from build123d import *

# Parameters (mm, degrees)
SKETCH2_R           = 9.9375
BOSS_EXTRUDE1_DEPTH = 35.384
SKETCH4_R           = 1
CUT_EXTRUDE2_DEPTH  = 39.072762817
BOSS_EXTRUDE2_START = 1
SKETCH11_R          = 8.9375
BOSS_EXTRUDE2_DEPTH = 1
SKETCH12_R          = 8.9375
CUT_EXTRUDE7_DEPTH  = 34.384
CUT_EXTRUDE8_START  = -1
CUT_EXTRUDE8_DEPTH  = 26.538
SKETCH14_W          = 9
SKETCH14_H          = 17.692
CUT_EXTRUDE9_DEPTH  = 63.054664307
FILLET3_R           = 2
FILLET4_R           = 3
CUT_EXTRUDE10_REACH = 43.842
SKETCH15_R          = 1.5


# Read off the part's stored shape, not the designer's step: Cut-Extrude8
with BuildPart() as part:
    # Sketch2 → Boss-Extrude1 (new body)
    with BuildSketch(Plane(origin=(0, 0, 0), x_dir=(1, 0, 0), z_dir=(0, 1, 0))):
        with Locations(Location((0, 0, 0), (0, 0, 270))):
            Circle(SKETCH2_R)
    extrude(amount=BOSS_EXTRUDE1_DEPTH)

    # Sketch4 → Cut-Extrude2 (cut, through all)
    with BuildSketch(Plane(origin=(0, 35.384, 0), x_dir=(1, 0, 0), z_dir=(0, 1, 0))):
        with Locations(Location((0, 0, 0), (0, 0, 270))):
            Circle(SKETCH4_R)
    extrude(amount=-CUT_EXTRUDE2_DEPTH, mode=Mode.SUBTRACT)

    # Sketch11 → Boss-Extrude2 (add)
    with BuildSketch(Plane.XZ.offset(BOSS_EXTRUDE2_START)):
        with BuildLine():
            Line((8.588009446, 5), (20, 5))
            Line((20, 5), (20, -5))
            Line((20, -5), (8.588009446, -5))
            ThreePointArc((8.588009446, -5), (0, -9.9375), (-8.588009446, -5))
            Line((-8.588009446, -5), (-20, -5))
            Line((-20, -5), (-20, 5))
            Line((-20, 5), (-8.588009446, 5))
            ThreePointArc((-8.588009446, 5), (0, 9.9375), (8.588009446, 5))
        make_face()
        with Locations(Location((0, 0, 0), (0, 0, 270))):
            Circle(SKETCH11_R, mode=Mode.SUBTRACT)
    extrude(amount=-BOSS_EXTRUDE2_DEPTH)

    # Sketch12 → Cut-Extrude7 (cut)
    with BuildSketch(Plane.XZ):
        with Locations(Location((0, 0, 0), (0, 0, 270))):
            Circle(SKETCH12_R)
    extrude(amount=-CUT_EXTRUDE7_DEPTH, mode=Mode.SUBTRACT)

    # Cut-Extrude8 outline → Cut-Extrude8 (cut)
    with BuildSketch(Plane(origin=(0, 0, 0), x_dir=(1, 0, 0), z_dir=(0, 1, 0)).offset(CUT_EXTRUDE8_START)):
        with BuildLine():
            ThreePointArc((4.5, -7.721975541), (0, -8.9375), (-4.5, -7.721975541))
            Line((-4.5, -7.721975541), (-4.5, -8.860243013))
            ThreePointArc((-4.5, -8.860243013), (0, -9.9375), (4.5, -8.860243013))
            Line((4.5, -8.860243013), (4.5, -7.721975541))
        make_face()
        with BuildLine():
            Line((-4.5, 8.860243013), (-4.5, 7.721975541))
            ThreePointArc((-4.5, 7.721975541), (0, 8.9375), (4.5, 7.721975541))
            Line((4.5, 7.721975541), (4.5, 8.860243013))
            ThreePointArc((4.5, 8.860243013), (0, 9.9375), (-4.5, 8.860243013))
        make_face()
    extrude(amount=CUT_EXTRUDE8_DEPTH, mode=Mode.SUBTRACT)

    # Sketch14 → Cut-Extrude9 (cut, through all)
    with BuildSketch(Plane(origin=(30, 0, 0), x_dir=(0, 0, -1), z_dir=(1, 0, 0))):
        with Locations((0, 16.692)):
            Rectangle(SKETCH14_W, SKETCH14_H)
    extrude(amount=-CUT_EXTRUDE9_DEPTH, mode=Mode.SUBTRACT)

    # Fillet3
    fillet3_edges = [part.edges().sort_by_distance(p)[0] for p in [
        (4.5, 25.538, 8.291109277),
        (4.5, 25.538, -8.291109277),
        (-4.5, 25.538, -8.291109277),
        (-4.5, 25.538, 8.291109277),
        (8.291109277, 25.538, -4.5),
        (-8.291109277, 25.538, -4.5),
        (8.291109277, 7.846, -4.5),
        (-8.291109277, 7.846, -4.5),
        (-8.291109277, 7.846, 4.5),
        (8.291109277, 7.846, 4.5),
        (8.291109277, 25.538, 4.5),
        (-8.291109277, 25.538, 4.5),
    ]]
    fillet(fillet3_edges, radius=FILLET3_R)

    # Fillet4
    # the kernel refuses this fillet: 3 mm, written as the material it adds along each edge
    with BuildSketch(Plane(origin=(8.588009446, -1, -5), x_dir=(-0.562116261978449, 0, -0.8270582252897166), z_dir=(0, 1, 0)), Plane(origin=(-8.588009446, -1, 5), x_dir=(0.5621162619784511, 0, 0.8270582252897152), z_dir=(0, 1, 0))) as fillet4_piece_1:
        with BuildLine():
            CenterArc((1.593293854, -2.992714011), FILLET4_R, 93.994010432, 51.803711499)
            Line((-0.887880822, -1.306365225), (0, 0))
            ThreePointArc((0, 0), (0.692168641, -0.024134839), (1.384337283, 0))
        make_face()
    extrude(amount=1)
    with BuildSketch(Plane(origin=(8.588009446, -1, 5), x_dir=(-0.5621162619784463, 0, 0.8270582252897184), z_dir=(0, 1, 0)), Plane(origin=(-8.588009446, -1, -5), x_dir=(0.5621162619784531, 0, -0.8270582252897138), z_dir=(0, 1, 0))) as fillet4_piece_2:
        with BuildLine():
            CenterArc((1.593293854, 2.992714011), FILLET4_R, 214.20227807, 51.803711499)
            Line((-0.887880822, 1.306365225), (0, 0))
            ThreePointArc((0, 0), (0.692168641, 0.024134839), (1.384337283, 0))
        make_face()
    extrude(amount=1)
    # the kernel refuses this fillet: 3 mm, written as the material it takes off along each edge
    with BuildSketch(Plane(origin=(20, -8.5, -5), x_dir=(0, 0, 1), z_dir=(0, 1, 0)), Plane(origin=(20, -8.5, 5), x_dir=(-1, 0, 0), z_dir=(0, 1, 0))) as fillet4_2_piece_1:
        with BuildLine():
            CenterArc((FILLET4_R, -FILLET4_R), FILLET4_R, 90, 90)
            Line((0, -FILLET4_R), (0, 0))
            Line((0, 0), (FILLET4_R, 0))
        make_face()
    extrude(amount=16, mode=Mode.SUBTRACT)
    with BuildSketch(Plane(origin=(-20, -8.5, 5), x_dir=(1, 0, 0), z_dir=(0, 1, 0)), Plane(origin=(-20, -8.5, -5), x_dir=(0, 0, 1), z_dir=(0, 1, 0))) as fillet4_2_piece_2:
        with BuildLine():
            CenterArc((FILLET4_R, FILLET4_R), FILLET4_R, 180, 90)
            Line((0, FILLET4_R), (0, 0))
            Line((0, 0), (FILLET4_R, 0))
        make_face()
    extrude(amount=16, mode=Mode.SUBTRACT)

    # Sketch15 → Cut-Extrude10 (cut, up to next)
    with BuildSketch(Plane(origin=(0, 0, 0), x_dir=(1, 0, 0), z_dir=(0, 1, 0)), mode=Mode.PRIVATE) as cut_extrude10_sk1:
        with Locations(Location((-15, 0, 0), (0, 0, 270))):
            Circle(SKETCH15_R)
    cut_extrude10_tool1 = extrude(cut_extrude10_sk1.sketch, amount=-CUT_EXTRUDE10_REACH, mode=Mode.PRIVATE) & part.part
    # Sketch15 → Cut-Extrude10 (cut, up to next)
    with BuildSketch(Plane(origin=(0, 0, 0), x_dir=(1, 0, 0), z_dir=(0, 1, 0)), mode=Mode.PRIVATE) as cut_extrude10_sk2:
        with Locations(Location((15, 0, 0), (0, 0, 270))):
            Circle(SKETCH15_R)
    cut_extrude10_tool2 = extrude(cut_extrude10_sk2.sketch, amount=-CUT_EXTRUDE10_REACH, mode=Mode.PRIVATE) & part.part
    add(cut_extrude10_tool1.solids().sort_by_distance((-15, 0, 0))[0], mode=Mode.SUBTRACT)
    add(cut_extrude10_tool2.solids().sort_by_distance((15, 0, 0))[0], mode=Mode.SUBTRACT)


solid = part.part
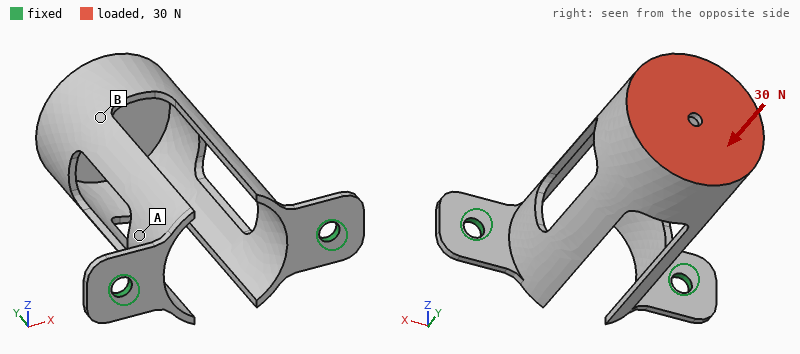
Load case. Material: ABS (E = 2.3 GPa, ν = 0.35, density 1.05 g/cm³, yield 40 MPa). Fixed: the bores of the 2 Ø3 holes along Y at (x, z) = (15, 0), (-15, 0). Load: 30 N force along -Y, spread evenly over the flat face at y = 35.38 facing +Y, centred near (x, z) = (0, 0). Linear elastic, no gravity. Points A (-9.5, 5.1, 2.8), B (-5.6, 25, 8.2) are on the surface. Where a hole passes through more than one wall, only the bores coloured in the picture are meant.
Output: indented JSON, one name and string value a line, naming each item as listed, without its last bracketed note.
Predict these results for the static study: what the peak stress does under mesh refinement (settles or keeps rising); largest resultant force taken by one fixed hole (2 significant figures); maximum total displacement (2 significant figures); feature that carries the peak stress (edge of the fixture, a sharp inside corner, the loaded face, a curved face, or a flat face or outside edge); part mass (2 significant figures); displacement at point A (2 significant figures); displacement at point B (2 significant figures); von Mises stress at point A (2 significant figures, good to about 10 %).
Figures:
{
  "what the peak stress does under mesh refinement": "keeps rising",
  "largest resultant force taken by one fixed hole": "15 N",
  "maximum total displacement": "0.27 mm",
  "feature that carries the peak stress": "edge of the fixture",
  "part mass": "1.9 g",
  "displacement at point A": "0.17 mm",
  "displacement at point B": "0.19 mm",
  "von Mises stress at point A": "4.4 MPa"
}
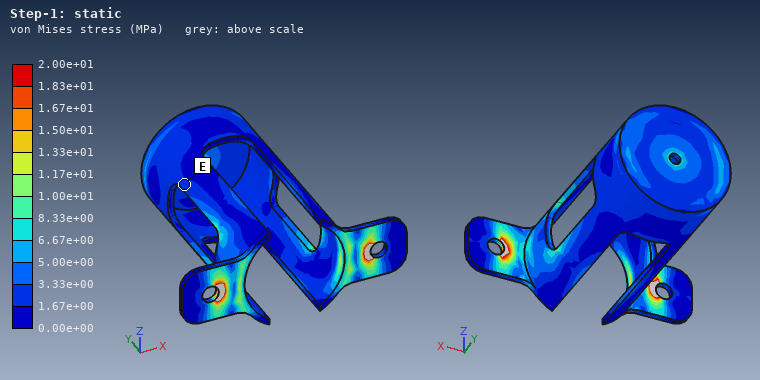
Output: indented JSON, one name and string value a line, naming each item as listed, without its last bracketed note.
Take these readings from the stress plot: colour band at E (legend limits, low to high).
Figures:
{
  "colour band at E": "1.67e+00 to 3.33e+00 MPa"
}
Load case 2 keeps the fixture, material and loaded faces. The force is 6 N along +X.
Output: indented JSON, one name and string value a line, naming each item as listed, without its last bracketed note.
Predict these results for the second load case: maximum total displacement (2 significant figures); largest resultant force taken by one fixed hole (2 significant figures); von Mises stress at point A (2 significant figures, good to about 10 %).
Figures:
{
  "maximum total displacement": "0.40 mm",
  "largest resultant force taken by one fixed hole": "9.7 N",
  "von Mises stress at point A": "2.8 MPa"
}
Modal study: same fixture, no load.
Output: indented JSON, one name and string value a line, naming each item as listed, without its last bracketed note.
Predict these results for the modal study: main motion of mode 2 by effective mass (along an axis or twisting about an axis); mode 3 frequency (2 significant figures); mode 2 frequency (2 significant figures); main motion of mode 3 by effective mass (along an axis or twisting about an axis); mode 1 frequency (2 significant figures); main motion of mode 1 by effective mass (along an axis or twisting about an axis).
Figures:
{
  "main motion of mode 2 by effective mass": "along X",
  "mode 3 frequency": "1100 Hz",
  "mode 2 frequency": "630 Hz",
  "main motion of mode 3 by effective mass": "twisting about Y",
  "mode 1 frequency": "190 Hz",
  "main motion of mode 1 by effective mass": "along Z"
}
